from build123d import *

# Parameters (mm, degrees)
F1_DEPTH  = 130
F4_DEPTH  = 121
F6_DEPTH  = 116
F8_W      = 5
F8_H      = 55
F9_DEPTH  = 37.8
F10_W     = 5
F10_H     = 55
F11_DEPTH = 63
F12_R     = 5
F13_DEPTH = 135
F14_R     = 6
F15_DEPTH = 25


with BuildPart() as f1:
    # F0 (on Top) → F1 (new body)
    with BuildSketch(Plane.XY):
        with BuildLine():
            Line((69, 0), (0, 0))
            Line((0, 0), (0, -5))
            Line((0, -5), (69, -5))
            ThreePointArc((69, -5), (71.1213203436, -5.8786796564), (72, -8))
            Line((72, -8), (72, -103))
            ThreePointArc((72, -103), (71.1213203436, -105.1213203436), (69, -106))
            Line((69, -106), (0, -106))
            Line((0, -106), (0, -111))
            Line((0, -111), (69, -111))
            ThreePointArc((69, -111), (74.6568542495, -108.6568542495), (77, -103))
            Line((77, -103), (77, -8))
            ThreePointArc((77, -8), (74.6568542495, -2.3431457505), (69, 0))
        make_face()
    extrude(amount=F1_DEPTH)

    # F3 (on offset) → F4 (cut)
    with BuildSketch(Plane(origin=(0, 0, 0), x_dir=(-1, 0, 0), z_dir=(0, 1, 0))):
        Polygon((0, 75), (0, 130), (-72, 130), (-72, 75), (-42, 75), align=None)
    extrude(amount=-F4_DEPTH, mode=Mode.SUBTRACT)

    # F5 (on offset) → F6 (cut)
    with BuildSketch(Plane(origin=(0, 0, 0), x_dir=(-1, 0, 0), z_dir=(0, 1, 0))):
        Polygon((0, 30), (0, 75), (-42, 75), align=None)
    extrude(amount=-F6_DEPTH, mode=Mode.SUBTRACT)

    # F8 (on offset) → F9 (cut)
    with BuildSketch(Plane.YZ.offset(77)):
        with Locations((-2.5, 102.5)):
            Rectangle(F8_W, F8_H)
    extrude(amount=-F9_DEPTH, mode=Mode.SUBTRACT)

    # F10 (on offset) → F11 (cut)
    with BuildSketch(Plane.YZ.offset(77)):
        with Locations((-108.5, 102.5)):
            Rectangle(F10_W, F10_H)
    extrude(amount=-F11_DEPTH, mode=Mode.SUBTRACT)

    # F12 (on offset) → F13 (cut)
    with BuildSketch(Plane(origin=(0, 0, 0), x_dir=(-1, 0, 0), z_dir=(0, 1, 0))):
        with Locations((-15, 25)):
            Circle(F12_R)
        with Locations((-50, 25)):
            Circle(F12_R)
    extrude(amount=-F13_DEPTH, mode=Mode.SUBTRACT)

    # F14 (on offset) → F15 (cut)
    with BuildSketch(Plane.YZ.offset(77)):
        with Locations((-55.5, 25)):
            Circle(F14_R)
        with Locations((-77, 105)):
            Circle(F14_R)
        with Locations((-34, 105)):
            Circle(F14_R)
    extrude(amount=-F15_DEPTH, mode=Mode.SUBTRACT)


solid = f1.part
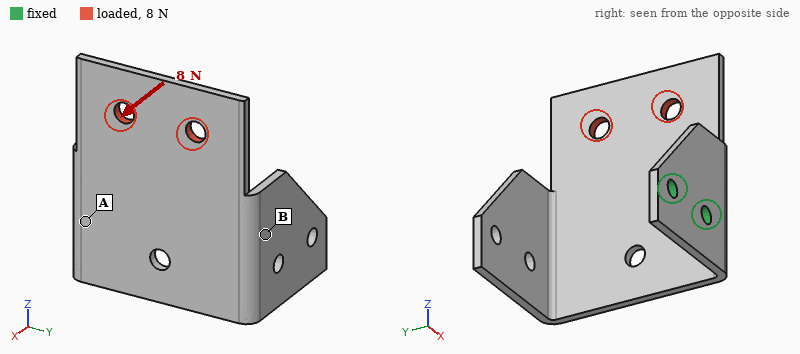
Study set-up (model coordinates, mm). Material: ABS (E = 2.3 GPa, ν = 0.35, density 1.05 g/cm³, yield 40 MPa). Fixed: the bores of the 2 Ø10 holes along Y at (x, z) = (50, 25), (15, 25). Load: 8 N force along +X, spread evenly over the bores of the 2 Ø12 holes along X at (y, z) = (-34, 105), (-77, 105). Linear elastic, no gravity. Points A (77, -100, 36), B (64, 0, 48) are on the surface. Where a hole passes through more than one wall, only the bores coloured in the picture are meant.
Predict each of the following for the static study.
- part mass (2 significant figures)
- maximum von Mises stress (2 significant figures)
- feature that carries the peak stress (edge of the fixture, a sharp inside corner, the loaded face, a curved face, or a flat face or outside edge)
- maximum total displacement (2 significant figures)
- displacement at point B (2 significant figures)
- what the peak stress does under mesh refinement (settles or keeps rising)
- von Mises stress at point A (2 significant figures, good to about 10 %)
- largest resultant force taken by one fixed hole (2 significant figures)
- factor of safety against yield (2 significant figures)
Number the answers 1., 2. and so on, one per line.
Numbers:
1. 110 g
2. 6.6 MPa
3. a curved face
4. 1.9 mm
5. 1.3 mm
6. settles
7. 1.2 MPa
8. 16 N
9. 6.0
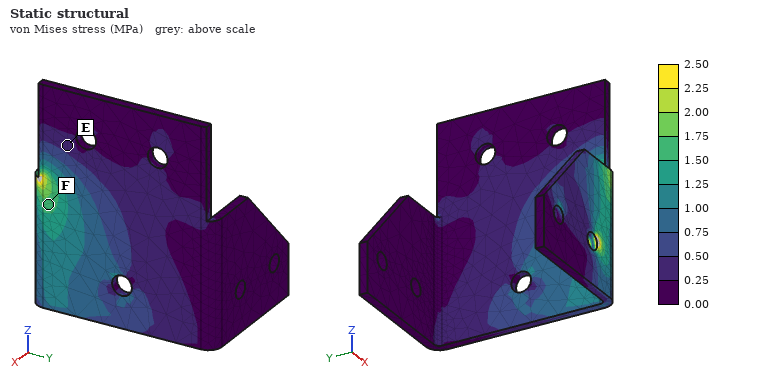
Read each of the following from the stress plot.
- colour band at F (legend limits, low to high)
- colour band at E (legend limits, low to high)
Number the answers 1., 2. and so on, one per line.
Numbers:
1. 1.50 to 1.75 MPa
2. 0.25 to 0.50 MPa
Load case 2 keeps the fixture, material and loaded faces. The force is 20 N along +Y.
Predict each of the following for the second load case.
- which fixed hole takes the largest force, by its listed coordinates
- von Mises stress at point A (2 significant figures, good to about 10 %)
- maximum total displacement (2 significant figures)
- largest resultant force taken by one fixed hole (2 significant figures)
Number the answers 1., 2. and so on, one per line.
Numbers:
1. (50, 25)
2. 1.1 MPa
3. 2.1 mm
4. 26 N
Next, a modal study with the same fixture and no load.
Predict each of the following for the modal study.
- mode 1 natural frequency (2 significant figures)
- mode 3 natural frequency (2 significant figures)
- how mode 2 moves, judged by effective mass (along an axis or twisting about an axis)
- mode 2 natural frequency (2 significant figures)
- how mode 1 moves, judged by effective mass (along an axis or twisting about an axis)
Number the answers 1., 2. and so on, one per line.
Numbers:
1. 41 Hz
2. 110 Hz
3. along Z
4. 63 Hz
5. along X
